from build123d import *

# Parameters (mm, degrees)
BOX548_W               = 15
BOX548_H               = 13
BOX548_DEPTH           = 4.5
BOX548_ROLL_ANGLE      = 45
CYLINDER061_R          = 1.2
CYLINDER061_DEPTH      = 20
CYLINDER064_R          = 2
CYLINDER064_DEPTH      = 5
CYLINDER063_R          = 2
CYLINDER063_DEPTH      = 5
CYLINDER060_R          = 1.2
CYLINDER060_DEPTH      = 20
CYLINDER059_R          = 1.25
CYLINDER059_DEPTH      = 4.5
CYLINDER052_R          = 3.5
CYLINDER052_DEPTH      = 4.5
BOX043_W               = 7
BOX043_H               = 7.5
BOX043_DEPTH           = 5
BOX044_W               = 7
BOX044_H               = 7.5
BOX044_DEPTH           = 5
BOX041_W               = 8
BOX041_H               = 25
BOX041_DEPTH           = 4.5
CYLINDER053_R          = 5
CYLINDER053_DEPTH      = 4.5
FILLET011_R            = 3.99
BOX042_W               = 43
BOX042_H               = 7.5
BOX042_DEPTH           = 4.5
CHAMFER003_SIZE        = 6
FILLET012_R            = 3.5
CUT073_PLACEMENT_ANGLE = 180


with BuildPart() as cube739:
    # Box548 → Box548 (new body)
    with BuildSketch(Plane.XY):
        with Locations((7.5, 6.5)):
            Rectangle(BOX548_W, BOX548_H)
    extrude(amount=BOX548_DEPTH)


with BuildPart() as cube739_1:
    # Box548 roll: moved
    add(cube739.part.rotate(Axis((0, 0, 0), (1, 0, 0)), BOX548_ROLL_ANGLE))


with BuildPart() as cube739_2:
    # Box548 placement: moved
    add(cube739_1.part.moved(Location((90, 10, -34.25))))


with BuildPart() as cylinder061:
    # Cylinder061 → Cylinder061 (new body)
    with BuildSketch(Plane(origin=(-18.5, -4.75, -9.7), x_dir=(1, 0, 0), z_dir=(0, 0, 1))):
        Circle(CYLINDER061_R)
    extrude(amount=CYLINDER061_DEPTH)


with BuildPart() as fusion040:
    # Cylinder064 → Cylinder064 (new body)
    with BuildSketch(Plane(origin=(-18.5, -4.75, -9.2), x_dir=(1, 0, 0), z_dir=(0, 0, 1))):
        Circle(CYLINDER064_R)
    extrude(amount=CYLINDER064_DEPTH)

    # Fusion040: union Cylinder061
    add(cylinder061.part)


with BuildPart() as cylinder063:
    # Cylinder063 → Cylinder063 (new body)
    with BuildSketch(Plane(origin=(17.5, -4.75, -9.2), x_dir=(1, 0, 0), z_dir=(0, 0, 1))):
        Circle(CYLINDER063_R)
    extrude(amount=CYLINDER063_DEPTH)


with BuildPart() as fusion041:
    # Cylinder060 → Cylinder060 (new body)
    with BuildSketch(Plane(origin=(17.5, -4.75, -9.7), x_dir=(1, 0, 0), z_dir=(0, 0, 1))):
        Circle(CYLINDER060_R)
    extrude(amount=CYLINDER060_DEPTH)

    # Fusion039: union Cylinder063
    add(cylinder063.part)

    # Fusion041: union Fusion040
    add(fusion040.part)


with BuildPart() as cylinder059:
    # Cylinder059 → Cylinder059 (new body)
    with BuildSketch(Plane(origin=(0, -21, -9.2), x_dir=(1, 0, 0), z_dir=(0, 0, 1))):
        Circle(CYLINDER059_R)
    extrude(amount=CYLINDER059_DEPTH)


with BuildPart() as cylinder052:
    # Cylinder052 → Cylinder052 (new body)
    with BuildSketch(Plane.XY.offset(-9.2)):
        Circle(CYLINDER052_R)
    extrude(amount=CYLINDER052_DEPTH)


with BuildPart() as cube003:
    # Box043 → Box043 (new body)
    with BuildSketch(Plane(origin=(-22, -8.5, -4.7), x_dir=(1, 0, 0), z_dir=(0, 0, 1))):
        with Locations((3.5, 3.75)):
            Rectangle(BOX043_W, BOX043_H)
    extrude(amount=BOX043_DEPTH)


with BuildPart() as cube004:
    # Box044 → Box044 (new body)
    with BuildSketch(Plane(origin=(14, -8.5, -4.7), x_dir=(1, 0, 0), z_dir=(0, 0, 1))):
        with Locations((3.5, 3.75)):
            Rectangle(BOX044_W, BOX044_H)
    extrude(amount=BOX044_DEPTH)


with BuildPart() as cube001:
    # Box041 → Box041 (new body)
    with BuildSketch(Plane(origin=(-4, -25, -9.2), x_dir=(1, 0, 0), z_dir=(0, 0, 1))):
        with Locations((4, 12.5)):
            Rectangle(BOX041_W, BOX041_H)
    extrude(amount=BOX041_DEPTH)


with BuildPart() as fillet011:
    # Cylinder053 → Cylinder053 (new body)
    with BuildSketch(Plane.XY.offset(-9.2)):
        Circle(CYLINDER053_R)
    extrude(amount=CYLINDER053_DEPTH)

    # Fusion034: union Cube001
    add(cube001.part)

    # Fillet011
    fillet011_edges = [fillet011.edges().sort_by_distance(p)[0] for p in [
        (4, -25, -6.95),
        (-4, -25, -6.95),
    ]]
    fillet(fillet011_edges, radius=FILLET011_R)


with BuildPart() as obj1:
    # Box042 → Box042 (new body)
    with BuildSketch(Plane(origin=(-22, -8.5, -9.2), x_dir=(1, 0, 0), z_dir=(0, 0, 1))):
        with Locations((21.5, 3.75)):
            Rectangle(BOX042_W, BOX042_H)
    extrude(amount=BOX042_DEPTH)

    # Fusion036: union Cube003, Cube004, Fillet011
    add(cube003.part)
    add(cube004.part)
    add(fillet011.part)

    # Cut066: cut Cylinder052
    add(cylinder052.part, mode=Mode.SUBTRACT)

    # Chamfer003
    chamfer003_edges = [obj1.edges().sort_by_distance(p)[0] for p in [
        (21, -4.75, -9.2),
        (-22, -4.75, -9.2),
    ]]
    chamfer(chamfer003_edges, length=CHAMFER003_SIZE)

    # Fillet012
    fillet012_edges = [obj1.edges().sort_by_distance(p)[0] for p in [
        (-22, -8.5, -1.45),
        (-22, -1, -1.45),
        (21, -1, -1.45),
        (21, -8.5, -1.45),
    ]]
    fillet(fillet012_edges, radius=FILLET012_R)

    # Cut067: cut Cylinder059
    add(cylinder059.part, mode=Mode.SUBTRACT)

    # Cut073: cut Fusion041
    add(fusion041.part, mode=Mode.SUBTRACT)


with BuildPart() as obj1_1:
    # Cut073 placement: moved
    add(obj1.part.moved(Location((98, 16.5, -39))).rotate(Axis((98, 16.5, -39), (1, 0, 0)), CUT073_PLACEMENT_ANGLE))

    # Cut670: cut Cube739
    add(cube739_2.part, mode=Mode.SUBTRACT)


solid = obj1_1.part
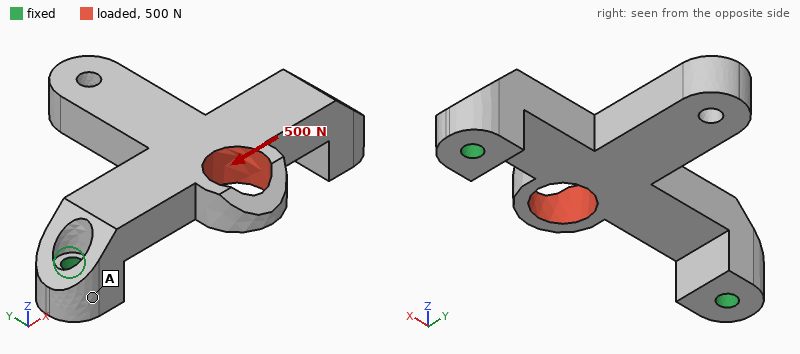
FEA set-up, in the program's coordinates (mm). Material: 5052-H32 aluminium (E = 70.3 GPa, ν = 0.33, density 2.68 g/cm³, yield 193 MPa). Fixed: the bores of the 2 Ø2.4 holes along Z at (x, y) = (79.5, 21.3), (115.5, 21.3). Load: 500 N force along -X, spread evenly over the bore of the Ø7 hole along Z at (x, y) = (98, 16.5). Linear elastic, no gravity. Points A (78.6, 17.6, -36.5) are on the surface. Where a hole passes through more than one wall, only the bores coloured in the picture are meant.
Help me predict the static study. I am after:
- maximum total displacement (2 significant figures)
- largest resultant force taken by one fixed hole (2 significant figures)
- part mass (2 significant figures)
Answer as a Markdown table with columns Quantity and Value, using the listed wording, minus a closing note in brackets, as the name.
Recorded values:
| Quantity | Value |
|---|---|
| maximum total displacement | 23 µm |
| largest resultant force taken by one fixed hole | 260 N |
| part mass | 5.7 g |
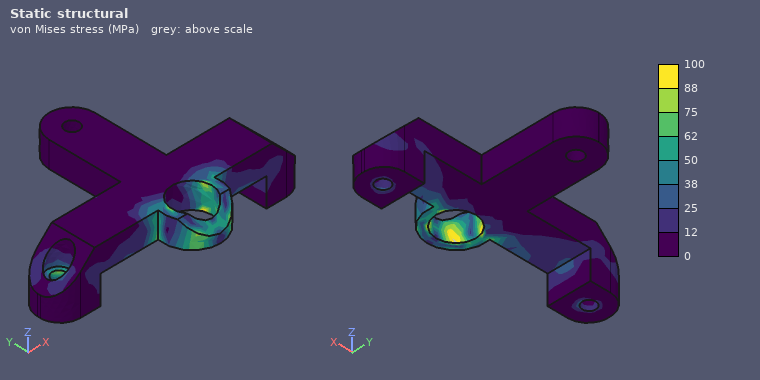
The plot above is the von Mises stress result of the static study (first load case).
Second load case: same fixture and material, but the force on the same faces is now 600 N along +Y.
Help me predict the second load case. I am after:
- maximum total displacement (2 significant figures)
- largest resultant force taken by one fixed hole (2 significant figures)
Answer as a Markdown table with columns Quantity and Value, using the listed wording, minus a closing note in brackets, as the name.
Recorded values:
| Quantity | Value |
|---|---|
| maximum total displacement | 32 µm |
| largest resultant force taken by one fixed hole | 310 N |
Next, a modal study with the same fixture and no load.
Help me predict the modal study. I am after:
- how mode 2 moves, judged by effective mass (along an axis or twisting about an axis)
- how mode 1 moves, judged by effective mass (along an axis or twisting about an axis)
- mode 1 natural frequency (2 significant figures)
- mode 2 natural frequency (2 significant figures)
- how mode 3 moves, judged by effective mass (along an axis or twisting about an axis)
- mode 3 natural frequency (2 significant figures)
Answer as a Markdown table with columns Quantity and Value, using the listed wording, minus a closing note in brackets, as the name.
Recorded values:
| Quantity | Value |
|---|---|
| how mode 2 moves, judged by effective mass | along Y |
| how mode 1 moves, judged by effective mass | along Z |
| mode 1 natural frequency | 5700 Hz |
| mode 2 natural frequency | 12 kHz |
| how mode 3 moves, judged by effective mass | along X |
| mode 3 natural frequency | 14 kHz |
